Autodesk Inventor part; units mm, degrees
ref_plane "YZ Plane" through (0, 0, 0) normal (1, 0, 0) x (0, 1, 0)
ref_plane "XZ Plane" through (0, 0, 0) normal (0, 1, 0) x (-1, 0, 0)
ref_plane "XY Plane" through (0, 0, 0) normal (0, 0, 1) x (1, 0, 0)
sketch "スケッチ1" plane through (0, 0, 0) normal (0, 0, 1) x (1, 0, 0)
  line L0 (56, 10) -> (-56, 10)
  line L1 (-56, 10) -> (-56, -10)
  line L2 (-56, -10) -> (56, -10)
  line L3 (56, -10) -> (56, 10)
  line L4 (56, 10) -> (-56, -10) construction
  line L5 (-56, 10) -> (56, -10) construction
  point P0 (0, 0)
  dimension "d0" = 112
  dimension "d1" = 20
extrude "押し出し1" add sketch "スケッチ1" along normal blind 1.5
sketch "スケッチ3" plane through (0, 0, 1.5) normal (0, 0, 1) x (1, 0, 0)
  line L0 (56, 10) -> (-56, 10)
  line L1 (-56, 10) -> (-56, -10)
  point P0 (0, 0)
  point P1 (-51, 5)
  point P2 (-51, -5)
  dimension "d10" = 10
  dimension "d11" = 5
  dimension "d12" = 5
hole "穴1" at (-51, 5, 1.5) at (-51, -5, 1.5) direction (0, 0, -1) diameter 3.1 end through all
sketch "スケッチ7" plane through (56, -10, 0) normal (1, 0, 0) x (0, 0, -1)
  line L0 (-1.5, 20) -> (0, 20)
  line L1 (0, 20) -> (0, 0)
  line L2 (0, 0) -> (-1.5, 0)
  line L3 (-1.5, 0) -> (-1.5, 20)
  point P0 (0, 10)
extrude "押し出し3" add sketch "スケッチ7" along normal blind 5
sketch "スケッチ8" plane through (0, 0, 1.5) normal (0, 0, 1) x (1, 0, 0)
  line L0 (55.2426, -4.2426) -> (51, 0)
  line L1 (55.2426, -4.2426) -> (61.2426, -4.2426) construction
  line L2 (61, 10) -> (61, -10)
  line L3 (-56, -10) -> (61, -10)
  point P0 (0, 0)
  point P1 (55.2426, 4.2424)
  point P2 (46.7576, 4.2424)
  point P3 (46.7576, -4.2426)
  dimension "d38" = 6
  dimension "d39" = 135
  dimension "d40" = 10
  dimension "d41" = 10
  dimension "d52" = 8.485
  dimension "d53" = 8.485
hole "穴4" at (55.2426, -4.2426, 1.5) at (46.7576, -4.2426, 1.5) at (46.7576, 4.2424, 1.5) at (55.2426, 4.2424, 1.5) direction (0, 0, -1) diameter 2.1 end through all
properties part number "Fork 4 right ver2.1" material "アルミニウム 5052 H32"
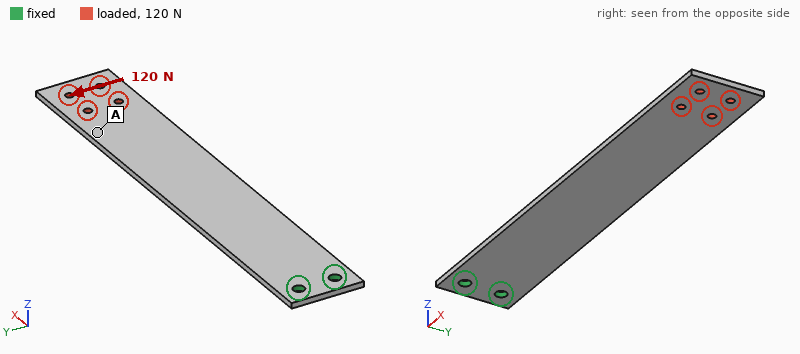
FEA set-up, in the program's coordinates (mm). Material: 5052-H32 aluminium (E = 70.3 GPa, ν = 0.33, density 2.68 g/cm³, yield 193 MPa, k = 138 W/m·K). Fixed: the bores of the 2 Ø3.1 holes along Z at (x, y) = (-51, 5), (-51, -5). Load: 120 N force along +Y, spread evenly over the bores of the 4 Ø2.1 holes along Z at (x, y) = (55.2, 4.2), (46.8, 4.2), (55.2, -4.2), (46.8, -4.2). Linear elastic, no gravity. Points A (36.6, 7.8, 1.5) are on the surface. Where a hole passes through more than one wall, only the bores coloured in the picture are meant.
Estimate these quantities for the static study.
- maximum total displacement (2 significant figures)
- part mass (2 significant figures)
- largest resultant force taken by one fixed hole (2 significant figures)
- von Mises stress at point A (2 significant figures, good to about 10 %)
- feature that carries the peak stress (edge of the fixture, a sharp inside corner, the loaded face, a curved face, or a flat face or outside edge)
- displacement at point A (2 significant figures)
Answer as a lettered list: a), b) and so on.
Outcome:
a) 0.75 mm
b) 9.3 g
c) 1.0 kN
d) 14 MPa
e) edge of the fixture
f) 0.52 mm
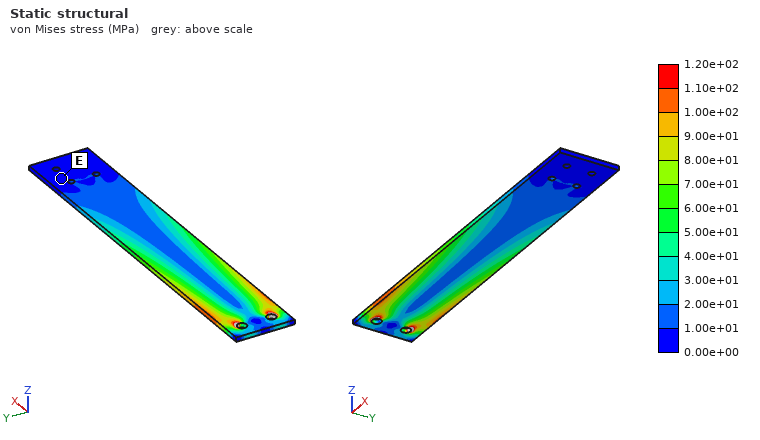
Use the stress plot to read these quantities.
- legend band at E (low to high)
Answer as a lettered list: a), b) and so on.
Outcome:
a) 0.00e+00 to 1.00e+01 MPa
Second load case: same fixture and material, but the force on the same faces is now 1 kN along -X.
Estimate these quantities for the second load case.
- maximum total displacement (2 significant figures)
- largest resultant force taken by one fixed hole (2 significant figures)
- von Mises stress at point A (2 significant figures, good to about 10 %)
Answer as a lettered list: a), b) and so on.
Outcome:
a) 50 µm
b) 500 N
c) 33 MPa
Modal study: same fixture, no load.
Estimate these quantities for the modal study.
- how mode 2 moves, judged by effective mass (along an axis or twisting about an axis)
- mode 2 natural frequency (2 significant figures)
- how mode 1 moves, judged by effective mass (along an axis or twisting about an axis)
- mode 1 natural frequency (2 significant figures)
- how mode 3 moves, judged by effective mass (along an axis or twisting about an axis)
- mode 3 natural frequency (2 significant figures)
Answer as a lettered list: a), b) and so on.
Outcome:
a) along Z
b) 640 Hz
c) along Z
d) 100 Hz
e) twisting about X
f) 1100 Hz
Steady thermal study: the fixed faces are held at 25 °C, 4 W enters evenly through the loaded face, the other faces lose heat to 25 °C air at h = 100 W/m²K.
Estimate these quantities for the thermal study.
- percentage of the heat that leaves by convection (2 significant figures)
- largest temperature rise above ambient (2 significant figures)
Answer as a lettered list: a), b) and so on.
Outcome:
a) 94 %
b) 23 K
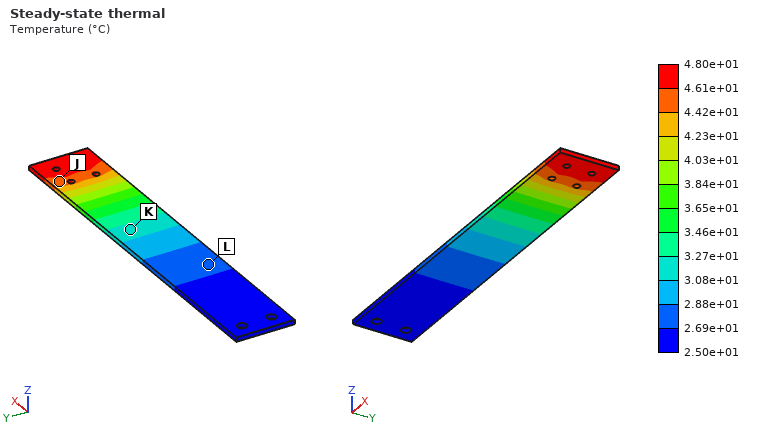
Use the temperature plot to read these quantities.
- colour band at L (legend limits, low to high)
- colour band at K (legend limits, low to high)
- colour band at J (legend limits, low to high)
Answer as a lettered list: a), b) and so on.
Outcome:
a) 2.69e+01 to 2.88e+01 °C
b) 3.08e+01 to 3.27e+01 °C
c) 4.42e+01 to 4.61e+01 °C
